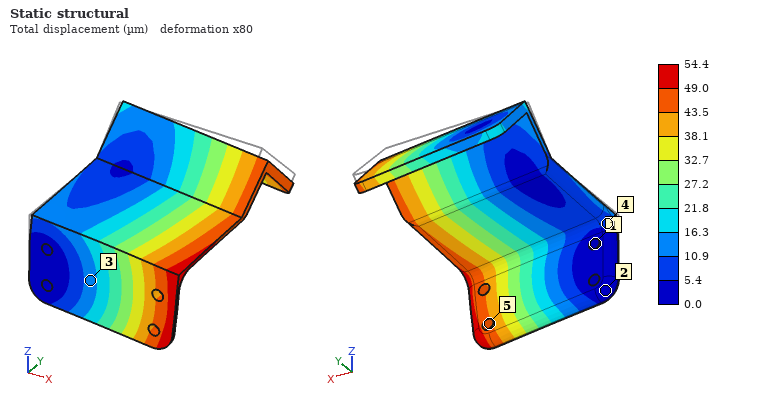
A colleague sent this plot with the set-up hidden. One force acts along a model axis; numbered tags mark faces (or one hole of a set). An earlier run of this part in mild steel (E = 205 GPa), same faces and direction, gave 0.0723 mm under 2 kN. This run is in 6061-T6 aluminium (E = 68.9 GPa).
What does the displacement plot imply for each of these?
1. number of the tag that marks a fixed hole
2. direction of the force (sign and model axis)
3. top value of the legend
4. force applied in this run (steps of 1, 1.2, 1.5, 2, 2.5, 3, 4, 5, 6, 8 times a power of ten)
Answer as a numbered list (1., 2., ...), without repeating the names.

1. 1
2. -Z
3. 54.4 µm
4. 500 N
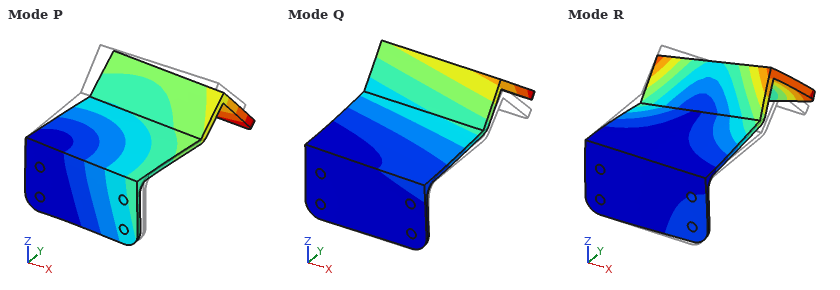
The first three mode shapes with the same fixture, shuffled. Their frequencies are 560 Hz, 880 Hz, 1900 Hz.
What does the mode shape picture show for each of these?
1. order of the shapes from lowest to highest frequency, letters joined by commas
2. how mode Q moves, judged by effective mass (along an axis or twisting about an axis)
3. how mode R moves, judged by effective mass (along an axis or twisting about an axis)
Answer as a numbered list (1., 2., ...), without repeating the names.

1. Q, P, R
2. along Z
3. twisting about Y
